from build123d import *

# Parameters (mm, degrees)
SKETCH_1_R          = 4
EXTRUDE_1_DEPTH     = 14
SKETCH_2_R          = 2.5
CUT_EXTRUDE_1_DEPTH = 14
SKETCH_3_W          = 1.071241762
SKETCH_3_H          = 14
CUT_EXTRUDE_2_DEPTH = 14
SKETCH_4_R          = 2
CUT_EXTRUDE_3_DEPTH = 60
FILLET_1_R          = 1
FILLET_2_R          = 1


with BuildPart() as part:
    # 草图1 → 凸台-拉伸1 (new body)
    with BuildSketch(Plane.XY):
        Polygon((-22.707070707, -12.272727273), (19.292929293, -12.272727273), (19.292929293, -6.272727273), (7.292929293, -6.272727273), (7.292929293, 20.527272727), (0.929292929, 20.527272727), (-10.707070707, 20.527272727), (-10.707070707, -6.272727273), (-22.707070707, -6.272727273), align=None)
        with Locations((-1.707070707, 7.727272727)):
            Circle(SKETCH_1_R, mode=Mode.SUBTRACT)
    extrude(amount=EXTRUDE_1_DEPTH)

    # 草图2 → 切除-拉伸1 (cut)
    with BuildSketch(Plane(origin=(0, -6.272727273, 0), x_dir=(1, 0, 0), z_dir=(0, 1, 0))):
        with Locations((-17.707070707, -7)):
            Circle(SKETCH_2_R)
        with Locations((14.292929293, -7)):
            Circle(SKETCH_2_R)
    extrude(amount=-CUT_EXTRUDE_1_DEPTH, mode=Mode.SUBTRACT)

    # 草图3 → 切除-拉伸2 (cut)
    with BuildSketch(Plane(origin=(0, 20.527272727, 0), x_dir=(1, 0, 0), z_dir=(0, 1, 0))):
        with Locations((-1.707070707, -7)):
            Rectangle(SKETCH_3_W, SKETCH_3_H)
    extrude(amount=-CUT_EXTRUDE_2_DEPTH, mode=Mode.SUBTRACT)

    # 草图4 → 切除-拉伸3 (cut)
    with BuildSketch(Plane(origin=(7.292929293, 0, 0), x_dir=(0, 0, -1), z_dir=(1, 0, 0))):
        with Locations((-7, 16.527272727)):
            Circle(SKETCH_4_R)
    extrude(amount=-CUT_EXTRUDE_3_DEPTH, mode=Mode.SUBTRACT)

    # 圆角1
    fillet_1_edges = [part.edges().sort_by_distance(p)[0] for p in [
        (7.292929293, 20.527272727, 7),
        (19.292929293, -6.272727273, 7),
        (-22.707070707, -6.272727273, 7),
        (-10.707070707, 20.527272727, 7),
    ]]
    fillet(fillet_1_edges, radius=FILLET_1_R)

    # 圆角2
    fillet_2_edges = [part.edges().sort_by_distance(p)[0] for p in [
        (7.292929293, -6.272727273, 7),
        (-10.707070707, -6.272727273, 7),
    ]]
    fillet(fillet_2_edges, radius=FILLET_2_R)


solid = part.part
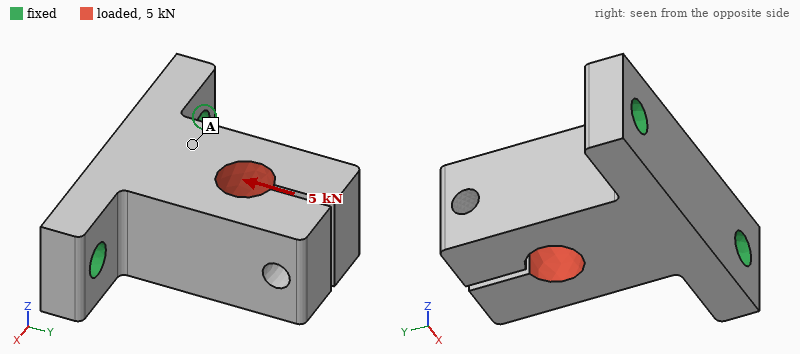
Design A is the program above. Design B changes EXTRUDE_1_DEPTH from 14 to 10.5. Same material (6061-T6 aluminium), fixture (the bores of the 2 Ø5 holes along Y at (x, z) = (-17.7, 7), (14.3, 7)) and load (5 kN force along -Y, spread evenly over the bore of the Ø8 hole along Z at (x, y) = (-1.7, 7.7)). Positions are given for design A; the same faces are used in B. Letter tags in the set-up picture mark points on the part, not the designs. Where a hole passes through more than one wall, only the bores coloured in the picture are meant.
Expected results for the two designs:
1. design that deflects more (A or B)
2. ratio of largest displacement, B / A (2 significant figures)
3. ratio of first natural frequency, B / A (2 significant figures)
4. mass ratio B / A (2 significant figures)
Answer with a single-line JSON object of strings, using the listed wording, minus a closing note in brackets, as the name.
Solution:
{"design that deflects more": "B", "ratio of largest displacement, B / A": "1.4", "ratio of first natural frequency, B / A": "0.91", "mass ratio B / A": "0.74"}
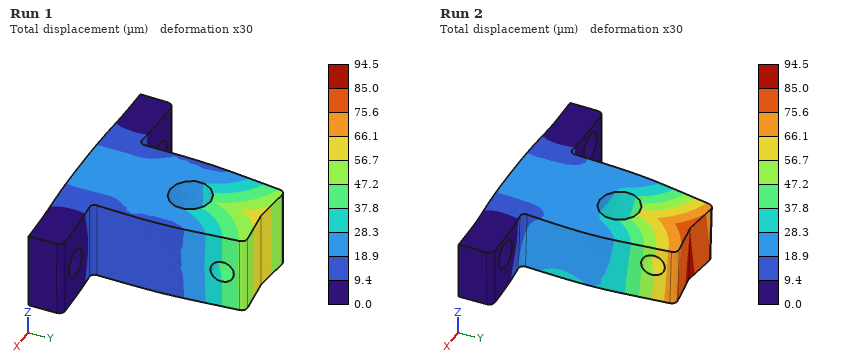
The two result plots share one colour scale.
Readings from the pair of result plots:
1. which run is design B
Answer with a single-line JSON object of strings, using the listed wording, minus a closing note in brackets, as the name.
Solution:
{"which run is design B": "Run 2"}
